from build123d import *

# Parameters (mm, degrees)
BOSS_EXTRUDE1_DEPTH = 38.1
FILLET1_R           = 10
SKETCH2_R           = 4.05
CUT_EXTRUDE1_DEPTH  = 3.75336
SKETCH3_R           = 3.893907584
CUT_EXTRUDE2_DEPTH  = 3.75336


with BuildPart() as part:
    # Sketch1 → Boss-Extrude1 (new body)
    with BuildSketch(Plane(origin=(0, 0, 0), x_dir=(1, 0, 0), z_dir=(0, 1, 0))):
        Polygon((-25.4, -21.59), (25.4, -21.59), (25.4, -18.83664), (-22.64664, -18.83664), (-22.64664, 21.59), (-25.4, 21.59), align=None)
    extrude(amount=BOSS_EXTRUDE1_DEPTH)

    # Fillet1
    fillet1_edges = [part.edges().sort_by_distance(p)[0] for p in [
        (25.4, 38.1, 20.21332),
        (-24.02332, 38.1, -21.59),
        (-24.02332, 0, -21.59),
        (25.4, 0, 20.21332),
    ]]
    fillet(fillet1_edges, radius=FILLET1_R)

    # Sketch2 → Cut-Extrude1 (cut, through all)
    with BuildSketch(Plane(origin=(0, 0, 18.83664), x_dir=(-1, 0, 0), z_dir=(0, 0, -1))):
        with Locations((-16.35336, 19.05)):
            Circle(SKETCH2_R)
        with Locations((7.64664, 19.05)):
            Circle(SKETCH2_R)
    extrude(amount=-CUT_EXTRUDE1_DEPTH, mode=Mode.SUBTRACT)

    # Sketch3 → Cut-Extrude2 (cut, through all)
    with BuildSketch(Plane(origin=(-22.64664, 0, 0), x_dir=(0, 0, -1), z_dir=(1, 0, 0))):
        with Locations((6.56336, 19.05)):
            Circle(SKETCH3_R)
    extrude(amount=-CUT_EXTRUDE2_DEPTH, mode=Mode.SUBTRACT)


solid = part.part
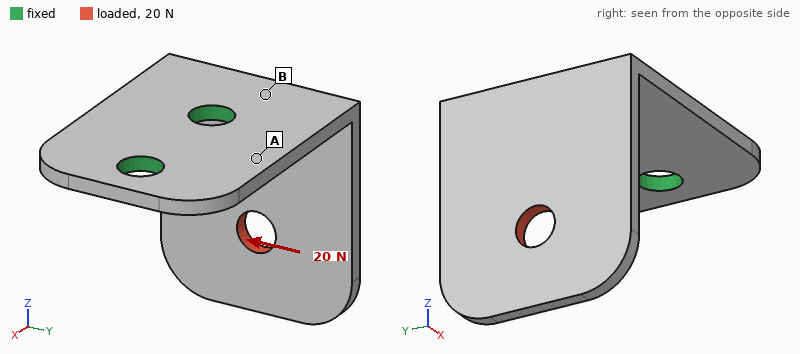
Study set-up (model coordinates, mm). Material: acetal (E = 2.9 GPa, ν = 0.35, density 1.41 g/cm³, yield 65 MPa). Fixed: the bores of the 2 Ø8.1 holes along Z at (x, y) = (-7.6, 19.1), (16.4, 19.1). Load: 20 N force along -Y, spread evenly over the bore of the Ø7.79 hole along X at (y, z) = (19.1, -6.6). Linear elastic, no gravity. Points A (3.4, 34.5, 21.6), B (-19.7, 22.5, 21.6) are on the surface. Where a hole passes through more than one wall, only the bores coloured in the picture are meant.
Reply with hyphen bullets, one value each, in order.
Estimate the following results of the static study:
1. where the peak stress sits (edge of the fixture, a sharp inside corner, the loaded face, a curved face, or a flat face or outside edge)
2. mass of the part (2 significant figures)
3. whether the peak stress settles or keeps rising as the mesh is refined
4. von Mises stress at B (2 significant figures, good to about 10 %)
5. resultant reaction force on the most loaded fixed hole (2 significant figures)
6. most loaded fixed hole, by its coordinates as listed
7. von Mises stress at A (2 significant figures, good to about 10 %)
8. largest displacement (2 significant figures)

- edge of the fixture
- 13 g
- keeps rising
- 5.7 MPa
- 28 N
- (-7.6, 19.1)
- 2.4 MPa
- 0.84 mm
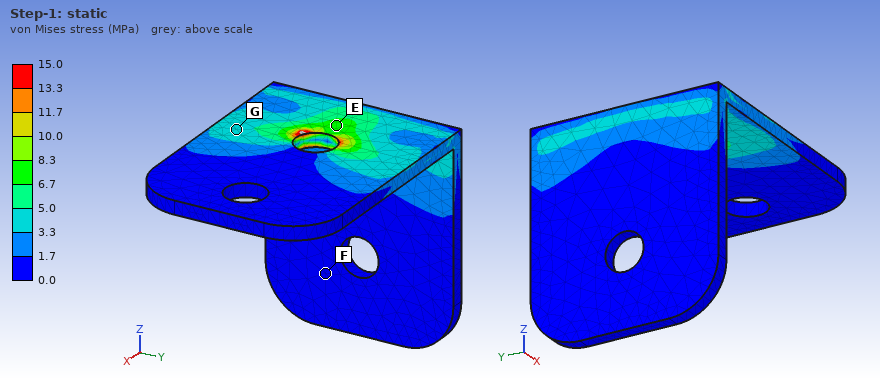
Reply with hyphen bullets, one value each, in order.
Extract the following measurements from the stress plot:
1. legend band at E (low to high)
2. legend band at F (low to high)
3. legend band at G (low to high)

- 6.7 to 8.3 MPa
- 0.0 to 1.7 MPa
- 3.3 to 5.0 MPa
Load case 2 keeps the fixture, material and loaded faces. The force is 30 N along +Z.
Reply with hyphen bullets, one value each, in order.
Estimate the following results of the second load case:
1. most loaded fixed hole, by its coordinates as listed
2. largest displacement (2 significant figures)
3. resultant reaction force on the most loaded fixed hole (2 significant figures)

- (-7.6, 19.1)
- 0.71 mm
- 33 N
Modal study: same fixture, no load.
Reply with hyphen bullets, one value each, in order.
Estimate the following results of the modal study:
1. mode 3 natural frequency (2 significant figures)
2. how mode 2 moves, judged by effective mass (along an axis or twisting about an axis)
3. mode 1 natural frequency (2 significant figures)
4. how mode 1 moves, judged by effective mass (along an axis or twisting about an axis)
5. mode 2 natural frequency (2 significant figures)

- 940 Hz
- along Y
- 260 Hz
- along X
- 420 Hz
